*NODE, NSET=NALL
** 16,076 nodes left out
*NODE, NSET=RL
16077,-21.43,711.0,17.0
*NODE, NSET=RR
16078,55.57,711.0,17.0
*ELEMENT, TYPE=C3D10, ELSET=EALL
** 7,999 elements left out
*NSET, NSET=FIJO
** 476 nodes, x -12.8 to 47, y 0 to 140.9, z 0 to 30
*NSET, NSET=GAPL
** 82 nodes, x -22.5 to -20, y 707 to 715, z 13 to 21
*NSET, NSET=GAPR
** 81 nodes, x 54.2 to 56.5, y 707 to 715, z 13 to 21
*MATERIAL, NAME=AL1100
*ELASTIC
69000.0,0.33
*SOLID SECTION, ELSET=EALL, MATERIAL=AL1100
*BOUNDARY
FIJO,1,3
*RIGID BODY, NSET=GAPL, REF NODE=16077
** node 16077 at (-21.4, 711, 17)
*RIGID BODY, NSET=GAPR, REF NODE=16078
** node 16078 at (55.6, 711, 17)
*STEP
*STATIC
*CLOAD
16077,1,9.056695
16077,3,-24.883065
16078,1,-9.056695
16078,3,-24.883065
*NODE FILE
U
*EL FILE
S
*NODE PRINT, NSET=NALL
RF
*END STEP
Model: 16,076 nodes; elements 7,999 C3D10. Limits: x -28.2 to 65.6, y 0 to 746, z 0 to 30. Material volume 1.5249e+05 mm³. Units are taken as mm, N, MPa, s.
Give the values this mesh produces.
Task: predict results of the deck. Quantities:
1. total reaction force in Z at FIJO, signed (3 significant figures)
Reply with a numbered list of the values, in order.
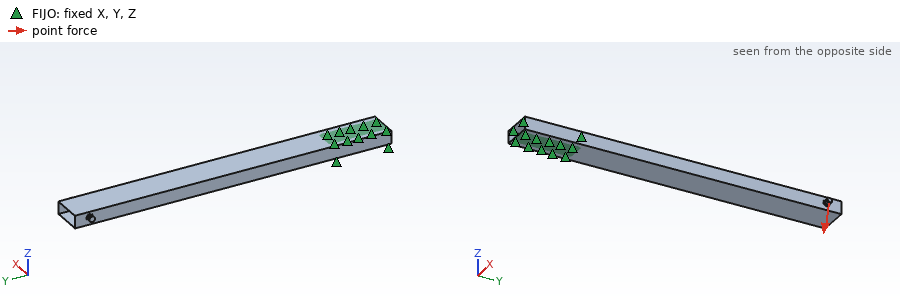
1. 49.8 N
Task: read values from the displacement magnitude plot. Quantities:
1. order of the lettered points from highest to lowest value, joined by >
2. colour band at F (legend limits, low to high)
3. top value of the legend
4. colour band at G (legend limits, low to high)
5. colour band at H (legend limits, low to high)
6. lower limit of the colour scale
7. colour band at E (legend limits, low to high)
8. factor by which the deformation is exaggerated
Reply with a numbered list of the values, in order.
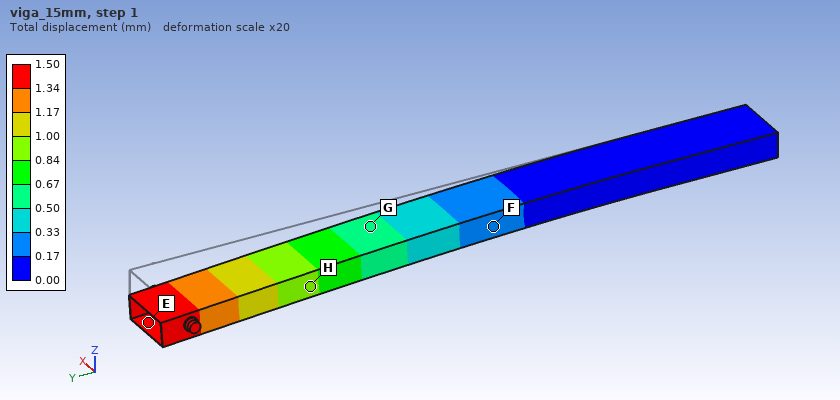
1. E > H > G > F
2. 0.17 to 0.33 mm
3. 1.50 mm
4. 0.50 to 0.67 mm
5. 0.84 to 1.00 mm
6. 0.00 mm
7. 1.34 to 1.50 mm
8. 20
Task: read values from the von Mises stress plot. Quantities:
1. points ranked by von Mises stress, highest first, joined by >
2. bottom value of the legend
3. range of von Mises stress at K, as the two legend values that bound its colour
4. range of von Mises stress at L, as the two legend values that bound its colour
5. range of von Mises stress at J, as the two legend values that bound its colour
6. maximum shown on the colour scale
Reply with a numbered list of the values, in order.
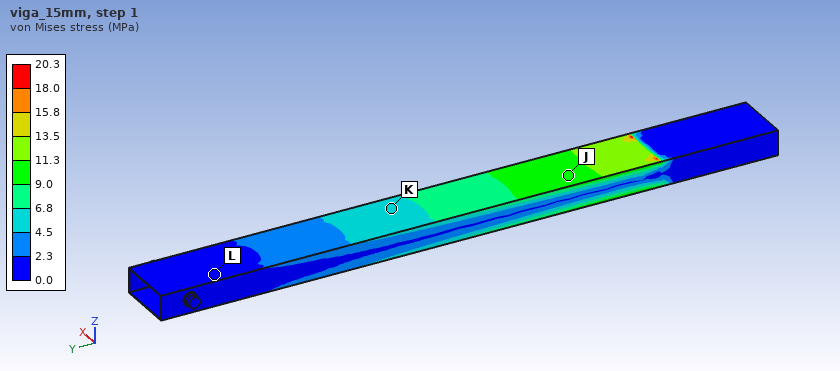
1. J > K > L
2. 0.0 MPa
3. 4.5 to 6.8 MPa
4. 0.0 to 2.3 MPa
5. 9.0 to 11.3 MPa
6. 20.3 MPa
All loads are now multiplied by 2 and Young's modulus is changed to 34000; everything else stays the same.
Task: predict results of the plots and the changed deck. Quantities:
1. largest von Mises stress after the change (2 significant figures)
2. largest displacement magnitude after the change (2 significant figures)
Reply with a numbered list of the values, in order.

1. 41 MPa
2. 6.1 mm
